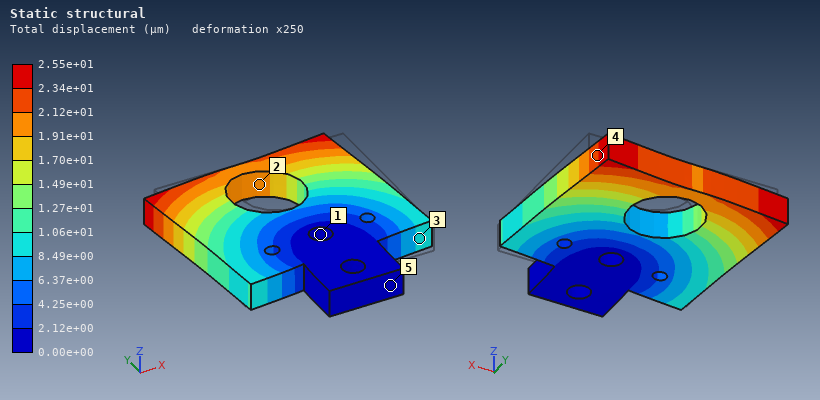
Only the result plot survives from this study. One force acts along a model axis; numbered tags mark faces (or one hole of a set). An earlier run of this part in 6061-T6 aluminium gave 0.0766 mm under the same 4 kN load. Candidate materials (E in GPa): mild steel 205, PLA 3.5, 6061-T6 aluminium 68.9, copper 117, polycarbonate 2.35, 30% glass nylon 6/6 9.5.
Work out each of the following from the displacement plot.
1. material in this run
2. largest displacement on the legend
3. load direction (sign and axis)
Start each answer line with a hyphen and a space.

- mild steel
- 2.55e+01 µm
- -X
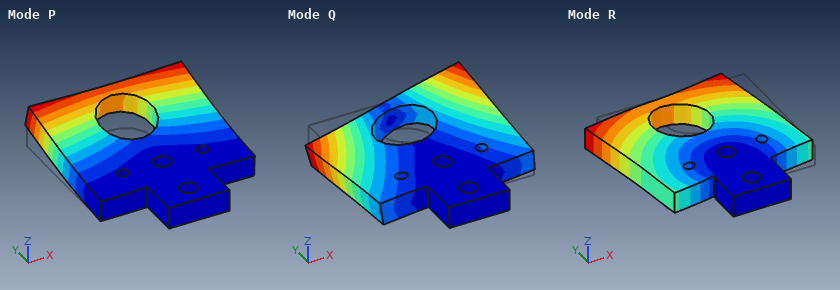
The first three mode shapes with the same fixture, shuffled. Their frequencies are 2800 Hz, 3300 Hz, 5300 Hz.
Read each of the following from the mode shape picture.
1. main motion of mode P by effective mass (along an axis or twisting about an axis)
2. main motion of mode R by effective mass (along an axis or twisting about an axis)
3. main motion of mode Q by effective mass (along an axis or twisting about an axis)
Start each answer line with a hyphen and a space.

- along Z
- along X
- twisting about Y
